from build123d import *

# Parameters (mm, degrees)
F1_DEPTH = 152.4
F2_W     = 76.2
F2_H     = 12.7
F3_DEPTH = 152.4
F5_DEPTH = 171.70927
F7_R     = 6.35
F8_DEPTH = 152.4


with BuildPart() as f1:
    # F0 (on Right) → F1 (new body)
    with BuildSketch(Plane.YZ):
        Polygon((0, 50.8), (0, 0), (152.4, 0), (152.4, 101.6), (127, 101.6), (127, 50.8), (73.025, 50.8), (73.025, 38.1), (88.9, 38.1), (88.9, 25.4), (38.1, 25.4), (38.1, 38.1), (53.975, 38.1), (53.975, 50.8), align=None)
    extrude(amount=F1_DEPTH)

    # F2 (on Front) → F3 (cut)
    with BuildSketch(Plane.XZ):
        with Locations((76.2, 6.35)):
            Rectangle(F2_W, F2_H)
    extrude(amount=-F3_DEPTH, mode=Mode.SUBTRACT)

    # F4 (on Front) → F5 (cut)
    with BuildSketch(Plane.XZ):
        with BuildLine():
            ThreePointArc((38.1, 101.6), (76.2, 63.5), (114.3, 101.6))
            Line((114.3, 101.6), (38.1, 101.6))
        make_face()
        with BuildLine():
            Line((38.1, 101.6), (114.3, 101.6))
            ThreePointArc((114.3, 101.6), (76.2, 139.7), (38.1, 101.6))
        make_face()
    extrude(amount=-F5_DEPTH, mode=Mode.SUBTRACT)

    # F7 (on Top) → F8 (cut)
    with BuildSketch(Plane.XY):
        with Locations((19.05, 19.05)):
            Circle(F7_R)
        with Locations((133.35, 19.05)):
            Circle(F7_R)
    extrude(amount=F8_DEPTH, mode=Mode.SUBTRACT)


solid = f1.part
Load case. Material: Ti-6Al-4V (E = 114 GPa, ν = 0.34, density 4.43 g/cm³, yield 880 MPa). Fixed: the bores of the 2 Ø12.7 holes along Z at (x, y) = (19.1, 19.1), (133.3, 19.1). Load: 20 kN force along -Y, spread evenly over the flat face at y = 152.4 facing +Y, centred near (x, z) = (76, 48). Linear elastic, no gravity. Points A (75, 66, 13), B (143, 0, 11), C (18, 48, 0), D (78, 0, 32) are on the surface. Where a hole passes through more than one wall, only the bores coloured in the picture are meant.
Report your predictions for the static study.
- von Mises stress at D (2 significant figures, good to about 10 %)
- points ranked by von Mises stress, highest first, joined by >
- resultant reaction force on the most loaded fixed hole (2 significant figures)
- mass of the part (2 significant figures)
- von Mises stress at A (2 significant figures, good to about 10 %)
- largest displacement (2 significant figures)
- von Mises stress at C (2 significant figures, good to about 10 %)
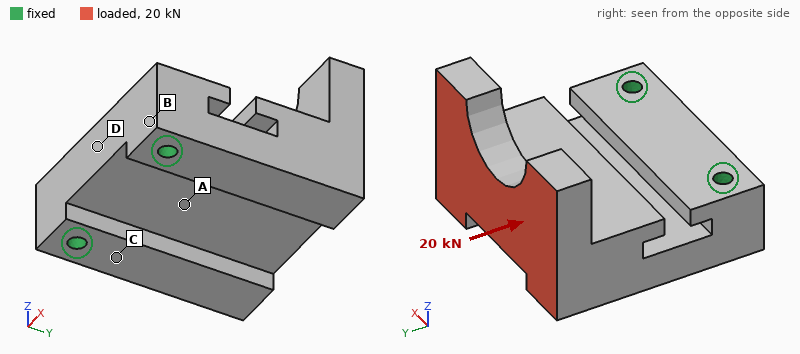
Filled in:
9.3 MPa
C > A > D > B
11 kN
4.5 kg
25 MPa
0.41 mm
59 MPa
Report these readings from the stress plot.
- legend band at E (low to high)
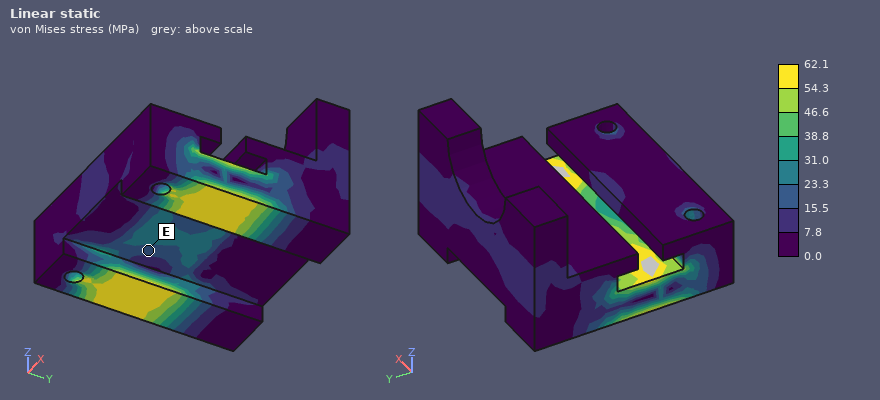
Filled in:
15.5 to 23.3 MPa
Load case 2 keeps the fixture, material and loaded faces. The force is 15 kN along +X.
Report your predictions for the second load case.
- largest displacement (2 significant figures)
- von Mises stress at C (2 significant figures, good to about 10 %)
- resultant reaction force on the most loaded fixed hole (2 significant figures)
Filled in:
76 µm
23 MPa
18 kN
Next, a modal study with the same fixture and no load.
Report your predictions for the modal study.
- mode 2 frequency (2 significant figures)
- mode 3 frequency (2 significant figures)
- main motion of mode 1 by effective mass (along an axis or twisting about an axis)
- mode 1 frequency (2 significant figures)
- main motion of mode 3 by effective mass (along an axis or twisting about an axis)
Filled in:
1500 Hz
2400 Hz
along Z
600 Hz
along X
